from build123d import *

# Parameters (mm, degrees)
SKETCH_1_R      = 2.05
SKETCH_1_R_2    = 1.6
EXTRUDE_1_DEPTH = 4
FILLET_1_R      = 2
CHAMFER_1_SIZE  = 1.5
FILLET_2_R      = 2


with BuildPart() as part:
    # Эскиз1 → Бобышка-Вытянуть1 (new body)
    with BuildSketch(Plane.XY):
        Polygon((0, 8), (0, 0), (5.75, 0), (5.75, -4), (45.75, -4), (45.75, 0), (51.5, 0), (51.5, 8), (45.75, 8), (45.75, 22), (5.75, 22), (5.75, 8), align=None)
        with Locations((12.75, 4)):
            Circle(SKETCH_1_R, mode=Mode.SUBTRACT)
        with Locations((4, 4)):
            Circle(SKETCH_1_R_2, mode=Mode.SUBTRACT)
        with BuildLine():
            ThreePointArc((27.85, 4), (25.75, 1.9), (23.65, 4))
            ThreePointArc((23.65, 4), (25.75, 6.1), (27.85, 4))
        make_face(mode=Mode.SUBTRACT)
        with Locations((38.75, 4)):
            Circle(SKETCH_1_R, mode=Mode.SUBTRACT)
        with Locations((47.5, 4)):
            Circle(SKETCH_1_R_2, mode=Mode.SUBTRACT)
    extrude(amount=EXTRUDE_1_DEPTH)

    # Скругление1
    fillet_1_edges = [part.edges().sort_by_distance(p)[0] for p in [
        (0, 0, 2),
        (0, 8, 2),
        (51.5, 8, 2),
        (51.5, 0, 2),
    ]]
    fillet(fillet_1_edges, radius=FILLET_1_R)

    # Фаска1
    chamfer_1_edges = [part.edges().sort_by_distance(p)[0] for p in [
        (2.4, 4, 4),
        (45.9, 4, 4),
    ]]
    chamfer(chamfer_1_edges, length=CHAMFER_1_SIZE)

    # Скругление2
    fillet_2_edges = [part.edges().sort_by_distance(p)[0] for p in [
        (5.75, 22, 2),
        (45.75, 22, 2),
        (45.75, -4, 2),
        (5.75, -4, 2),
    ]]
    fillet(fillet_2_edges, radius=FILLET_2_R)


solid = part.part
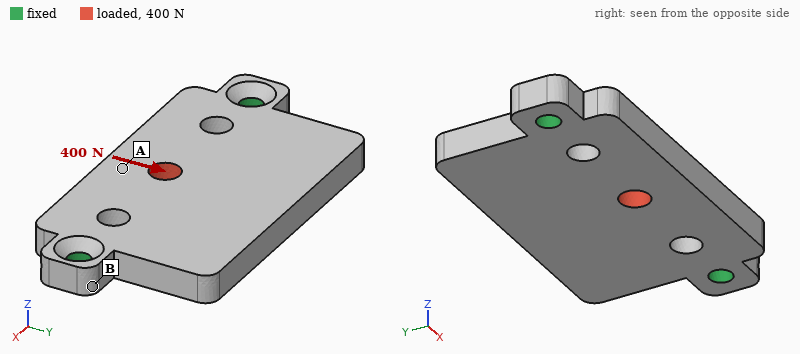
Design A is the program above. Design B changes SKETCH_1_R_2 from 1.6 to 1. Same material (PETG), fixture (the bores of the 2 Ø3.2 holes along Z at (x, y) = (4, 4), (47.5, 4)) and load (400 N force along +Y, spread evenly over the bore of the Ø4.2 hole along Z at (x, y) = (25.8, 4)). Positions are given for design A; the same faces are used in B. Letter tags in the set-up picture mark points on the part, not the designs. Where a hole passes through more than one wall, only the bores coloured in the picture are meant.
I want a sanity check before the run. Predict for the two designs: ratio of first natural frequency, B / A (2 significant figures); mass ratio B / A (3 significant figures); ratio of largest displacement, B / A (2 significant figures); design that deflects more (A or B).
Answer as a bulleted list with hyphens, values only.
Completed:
- 0.91
- 1.01
- 1.2
- B
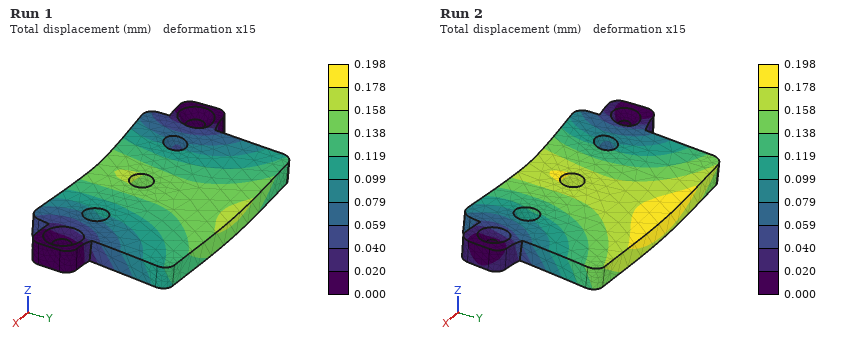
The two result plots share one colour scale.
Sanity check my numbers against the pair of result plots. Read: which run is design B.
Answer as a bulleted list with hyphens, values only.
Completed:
- Run 2
